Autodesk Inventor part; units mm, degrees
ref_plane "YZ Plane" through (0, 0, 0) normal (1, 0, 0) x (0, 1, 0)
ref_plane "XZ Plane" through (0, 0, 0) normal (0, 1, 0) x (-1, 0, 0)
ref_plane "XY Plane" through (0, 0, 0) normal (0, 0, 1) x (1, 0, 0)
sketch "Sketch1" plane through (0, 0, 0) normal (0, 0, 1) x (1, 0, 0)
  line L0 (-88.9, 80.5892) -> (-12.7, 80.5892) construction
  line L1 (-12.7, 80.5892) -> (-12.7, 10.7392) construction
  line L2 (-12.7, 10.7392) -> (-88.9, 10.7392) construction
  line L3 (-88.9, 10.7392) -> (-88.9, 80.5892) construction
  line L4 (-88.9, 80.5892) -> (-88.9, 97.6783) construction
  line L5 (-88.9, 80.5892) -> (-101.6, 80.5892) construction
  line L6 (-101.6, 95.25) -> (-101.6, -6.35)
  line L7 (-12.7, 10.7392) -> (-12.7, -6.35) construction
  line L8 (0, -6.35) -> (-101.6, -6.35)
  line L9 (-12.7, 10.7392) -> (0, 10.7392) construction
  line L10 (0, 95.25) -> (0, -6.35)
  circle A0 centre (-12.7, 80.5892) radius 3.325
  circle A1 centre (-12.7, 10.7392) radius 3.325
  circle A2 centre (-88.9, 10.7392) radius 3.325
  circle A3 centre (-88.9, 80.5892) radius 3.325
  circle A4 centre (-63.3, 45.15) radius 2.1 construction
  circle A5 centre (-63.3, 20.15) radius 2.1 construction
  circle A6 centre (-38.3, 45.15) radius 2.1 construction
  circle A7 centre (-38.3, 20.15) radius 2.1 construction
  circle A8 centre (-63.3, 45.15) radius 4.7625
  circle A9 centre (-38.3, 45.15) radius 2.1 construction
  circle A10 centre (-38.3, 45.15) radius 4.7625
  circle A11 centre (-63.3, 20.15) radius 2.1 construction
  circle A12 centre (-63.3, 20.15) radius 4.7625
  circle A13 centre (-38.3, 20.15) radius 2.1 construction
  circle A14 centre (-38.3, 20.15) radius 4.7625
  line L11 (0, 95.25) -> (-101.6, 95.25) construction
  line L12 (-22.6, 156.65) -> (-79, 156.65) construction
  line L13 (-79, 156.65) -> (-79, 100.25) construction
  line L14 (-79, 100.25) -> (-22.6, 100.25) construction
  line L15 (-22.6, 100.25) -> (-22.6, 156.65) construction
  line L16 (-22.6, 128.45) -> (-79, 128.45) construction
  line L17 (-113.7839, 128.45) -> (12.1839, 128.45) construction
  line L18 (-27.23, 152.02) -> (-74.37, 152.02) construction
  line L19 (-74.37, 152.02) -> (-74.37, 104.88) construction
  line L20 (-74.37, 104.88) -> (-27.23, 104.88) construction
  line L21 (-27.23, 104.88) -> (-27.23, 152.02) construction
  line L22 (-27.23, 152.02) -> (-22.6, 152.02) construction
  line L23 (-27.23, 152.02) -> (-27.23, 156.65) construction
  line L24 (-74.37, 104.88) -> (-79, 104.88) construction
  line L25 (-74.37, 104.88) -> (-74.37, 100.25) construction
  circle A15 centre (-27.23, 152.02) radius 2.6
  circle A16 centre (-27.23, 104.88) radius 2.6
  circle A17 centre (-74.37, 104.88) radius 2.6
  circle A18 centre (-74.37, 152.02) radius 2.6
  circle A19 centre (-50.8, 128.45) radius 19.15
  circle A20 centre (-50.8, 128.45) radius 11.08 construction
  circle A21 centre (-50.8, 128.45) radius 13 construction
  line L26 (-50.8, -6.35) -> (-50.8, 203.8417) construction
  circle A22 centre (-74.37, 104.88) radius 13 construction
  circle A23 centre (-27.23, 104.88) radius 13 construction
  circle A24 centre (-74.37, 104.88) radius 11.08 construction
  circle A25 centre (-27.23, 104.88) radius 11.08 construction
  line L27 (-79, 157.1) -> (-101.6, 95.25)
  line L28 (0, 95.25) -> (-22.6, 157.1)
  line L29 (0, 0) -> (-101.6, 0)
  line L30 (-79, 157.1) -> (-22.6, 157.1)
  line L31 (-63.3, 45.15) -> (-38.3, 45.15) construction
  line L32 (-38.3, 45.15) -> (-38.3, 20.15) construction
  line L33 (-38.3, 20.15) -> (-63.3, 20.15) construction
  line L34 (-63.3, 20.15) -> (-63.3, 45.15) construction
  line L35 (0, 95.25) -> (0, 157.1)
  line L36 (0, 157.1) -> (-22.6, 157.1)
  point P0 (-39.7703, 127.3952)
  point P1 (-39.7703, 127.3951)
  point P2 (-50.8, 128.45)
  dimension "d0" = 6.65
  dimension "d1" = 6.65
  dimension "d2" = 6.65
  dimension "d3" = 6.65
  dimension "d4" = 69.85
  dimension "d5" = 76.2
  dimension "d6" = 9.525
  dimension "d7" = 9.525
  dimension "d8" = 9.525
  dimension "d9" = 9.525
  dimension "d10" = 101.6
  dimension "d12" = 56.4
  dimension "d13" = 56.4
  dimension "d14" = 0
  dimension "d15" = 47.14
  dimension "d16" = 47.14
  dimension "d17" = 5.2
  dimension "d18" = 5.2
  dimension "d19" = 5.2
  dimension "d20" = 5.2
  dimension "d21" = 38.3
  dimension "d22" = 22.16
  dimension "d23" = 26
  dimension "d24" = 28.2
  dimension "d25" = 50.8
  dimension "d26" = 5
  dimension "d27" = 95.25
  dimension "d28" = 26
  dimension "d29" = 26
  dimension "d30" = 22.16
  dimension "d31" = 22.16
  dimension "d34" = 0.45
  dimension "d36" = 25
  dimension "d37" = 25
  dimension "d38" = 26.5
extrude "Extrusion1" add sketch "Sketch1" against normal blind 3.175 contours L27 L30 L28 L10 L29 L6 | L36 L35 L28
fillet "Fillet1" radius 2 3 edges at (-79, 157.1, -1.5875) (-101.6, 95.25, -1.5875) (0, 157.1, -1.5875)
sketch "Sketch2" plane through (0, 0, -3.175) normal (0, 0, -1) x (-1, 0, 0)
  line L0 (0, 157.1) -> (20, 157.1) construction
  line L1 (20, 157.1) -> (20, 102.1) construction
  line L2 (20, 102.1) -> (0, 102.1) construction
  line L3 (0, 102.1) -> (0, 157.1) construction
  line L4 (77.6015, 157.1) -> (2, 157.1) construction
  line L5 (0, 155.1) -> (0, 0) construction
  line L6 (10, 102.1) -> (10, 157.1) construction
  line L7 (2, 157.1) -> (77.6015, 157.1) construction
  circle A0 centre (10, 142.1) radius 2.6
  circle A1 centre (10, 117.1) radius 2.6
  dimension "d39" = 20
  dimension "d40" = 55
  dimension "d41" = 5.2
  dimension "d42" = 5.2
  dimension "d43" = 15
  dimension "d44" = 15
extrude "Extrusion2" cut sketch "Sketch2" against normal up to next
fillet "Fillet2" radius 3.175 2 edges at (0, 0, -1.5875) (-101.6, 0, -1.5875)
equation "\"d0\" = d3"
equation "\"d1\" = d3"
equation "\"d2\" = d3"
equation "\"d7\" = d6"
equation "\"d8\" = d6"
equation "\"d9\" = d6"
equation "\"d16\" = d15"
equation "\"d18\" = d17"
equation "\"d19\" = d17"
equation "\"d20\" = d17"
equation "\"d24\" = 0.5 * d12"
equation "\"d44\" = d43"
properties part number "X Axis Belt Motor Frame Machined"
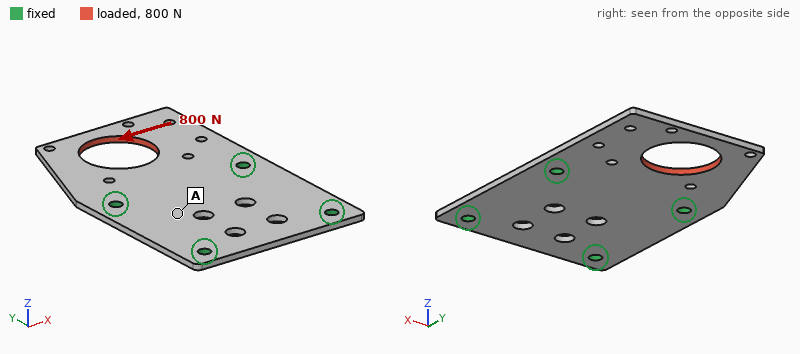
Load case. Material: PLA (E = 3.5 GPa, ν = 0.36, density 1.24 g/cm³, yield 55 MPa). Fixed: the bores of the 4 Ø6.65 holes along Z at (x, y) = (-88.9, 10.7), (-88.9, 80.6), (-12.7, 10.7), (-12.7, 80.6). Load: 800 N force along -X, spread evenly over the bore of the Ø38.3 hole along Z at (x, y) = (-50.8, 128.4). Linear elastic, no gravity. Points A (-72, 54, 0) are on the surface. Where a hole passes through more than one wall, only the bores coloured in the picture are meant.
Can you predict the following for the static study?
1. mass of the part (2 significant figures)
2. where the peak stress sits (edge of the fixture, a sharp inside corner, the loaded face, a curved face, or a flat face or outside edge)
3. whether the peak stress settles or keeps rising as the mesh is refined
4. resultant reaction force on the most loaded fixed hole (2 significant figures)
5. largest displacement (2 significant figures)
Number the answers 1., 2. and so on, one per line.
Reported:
1. 53 g
2. edge of the fixture
3. keeps rising
4. 590 N
5. 0.40 mm
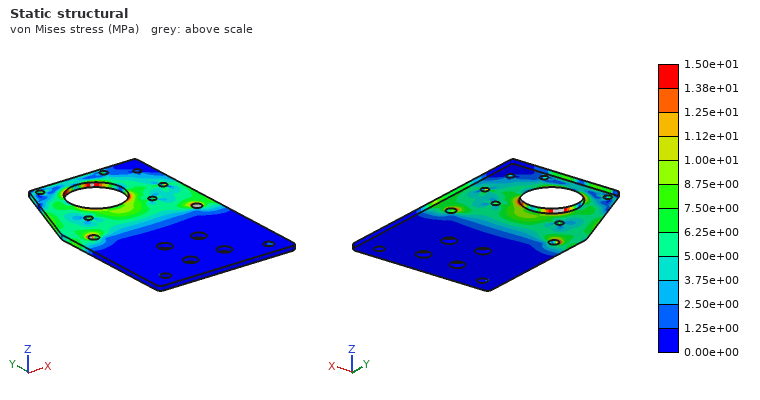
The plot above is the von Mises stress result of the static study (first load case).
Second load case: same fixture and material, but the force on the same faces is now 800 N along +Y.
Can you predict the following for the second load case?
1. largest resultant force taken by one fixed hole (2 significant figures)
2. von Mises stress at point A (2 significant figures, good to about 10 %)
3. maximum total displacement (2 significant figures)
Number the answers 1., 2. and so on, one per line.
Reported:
1. 340 N
2. 0.99 MPa
3. 0.15 mm
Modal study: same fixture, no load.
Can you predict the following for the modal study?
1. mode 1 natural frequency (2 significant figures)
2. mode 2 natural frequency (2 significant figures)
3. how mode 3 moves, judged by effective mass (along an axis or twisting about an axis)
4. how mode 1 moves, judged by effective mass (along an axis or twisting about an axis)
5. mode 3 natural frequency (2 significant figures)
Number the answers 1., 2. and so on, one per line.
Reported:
1. 160 Hz
2. 340 Hz
3. along Z
4. along Z
5. 770 Hz
